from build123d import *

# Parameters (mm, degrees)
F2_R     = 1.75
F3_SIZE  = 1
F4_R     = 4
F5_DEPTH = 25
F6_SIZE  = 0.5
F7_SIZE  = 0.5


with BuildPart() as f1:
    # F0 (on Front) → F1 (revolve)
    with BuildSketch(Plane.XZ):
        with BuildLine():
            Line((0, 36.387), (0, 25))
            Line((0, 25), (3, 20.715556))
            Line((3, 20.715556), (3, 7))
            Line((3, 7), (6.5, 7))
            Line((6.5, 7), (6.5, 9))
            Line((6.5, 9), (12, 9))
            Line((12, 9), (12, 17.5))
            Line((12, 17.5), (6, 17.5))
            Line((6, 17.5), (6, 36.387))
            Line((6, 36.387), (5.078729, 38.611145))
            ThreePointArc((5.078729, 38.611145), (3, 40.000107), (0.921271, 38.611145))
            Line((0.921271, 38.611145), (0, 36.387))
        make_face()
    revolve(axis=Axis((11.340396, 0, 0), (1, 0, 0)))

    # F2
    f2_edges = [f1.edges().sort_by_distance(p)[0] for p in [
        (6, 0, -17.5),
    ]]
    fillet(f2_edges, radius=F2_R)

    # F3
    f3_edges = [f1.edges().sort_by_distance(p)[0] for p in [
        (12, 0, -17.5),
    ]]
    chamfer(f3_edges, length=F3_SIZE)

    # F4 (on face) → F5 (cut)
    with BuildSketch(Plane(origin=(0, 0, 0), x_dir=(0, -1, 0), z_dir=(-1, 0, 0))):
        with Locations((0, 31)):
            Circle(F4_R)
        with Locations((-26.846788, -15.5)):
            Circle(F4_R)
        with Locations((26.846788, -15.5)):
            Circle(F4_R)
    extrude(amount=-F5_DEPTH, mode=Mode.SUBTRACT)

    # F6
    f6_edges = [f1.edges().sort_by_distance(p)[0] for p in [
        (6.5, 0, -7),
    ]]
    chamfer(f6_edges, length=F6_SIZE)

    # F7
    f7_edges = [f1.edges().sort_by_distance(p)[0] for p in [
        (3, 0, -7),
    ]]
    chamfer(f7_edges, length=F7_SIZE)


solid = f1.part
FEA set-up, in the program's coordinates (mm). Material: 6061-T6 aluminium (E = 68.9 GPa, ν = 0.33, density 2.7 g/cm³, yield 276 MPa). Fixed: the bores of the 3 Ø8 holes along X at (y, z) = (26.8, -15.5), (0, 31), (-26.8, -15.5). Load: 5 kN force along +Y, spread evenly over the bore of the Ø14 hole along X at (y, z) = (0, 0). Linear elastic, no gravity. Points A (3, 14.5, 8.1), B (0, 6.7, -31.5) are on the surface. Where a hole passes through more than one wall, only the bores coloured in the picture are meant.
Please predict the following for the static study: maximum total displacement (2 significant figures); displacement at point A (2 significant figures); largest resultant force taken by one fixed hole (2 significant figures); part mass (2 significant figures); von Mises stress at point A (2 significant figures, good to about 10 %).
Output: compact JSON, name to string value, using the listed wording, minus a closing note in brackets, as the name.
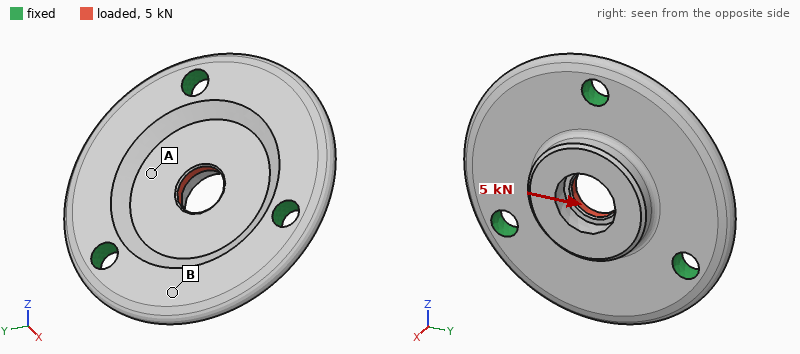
{"maximum total displacement": "11 µm", "displacement at point A": "7.7 µm", "largest resultant force taken by one fixed hole": "1.7 kN", "part mass": "72 g", "von Mises stress at point A": "24 MPa"}
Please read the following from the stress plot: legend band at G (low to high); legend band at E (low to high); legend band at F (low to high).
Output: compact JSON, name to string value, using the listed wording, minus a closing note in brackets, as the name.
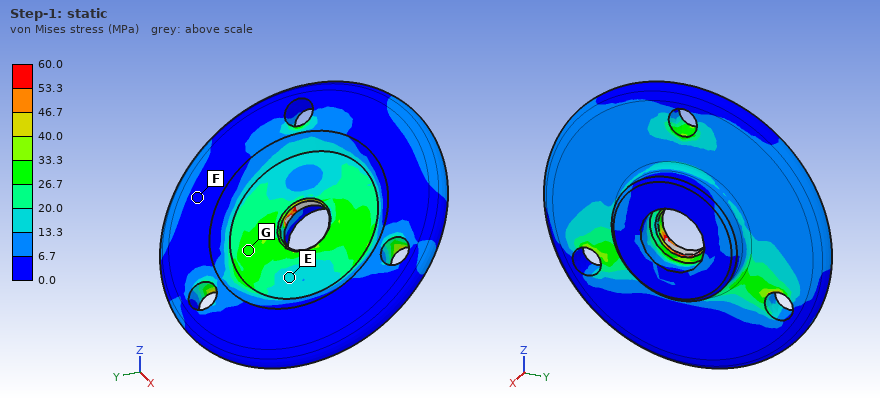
{"legend band at G": "26.7 to 33.3 MPa", "legend band at E": "13.3 to 20.0 MPa", "legend band at F": "0.0 to 6.7 MPa"}
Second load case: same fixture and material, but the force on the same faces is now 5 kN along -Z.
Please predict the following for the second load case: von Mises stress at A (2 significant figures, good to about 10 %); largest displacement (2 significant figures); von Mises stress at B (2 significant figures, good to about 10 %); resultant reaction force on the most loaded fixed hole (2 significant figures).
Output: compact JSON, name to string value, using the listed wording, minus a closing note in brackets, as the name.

{"von Mises stress at A": "18 MPa", "largest displacement": "12 µm", "von Mises stress at B": "6.8 MPa", "resultant reaction force on the most loaded fixed hole": "1.7 kN"}
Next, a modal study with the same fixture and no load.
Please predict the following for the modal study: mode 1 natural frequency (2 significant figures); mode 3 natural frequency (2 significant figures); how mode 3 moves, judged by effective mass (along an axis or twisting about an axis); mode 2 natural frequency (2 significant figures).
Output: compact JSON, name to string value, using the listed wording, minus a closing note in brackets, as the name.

{"mode 1 natural frequency": "7500 Hz", "mode 3 natural frequency": "7900 Hz", "how mode 3 moves, judged by effective mass": "along X", "mode 2 natural frequency": "7500 Hz"}
